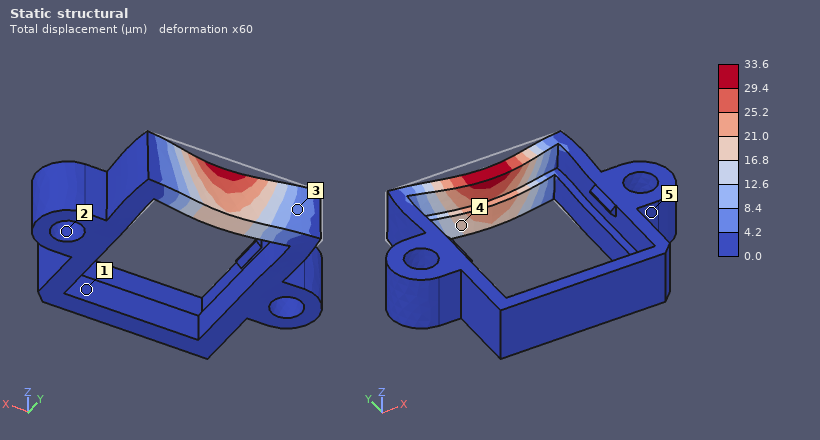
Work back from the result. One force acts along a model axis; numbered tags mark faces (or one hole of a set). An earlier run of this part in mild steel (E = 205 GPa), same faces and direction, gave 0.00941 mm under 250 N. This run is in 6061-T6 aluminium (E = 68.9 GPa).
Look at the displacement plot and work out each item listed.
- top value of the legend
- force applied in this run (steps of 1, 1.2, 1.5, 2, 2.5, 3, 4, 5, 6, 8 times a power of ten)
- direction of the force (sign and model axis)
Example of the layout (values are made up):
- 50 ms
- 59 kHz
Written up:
- 33.6 µm
- 300 N
- -Y
